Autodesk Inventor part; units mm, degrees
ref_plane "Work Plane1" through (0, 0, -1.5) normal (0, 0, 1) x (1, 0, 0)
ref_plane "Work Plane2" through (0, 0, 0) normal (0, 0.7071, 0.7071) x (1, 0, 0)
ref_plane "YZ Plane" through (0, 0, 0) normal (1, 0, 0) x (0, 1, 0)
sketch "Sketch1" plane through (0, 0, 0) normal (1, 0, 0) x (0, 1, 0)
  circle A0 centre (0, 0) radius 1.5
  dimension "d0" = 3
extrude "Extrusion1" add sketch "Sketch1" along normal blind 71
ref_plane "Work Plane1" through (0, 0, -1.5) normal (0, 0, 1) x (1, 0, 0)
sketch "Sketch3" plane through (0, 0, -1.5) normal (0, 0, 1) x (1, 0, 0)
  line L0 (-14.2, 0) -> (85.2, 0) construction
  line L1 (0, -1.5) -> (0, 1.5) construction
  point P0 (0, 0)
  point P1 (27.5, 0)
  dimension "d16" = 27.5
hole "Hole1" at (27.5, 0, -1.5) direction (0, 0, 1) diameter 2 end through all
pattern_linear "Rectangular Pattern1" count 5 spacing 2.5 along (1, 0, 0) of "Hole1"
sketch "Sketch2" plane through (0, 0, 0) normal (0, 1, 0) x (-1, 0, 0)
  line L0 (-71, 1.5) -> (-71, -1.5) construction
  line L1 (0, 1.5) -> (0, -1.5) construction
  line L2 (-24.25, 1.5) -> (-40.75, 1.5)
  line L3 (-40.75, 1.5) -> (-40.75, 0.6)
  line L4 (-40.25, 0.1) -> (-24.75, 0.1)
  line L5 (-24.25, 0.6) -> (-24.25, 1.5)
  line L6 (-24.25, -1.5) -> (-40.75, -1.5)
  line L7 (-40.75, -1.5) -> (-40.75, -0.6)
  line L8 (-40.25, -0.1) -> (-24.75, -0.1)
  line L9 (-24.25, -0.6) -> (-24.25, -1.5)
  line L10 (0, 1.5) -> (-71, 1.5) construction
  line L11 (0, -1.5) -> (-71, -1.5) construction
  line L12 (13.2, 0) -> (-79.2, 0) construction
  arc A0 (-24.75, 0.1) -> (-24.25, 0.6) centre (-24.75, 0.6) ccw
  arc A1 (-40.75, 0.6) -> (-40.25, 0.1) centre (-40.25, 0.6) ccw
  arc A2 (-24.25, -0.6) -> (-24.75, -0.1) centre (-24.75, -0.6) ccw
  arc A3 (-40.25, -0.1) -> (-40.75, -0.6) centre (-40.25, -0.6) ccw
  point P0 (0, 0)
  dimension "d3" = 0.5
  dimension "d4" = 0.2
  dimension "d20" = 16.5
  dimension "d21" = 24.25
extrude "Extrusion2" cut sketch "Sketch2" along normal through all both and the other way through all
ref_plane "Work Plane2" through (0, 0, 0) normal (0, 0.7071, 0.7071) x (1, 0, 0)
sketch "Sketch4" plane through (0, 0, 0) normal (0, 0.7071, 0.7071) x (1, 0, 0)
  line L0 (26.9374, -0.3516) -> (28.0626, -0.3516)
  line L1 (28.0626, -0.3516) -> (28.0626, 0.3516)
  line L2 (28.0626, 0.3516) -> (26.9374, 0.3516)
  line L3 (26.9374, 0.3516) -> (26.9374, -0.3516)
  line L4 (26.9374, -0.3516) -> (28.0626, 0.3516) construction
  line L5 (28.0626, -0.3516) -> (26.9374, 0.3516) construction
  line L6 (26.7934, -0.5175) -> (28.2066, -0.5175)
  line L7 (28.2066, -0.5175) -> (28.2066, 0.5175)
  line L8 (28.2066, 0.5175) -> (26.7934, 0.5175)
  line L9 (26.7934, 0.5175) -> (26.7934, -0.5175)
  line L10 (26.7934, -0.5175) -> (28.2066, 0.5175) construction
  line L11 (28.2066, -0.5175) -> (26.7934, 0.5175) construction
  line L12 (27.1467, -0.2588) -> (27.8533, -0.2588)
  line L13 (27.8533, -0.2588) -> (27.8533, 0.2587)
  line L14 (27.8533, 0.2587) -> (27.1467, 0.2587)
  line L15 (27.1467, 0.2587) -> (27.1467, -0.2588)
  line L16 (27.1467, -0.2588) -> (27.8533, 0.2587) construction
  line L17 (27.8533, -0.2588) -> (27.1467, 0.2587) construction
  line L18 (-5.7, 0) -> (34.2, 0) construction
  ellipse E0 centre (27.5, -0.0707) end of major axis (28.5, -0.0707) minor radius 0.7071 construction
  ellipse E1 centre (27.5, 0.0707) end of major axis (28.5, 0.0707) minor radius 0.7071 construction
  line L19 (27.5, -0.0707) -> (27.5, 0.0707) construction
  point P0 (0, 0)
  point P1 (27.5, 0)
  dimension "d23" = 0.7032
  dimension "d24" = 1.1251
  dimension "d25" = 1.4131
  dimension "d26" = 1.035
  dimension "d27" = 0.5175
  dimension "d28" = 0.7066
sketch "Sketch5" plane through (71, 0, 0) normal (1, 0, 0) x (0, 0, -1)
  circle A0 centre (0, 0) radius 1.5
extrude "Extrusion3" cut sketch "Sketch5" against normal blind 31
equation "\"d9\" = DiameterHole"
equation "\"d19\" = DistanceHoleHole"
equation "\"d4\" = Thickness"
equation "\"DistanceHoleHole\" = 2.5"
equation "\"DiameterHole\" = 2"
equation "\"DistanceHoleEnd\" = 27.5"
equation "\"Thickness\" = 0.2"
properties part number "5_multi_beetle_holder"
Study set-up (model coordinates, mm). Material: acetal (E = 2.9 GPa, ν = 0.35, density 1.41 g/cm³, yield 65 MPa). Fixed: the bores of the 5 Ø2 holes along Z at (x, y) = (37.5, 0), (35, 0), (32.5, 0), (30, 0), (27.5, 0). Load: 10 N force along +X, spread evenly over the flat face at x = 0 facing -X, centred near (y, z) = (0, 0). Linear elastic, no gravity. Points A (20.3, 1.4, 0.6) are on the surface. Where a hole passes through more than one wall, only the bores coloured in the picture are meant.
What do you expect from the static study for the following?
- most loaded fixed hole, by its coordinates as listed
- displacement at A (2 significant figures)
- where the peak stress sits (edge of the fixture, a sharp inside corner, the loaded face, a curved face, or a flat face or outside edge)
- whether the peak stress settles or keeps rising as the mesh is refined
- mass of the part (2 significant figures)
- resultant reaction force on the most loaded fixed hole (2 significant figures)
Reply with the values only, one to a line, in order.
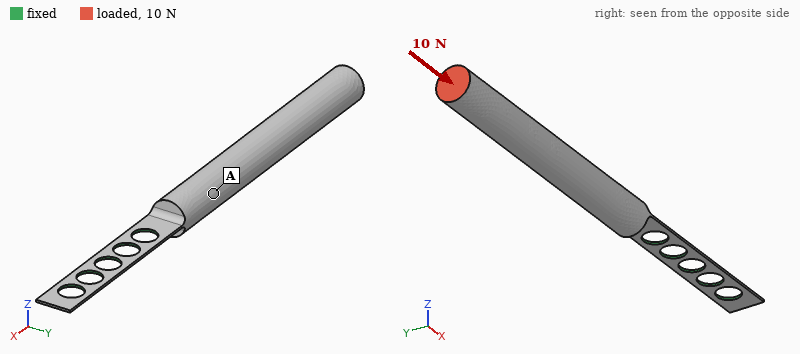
(27.5, 0)
17 µm
edge of the fixture
keeps rising
0.25 g
9.8 N
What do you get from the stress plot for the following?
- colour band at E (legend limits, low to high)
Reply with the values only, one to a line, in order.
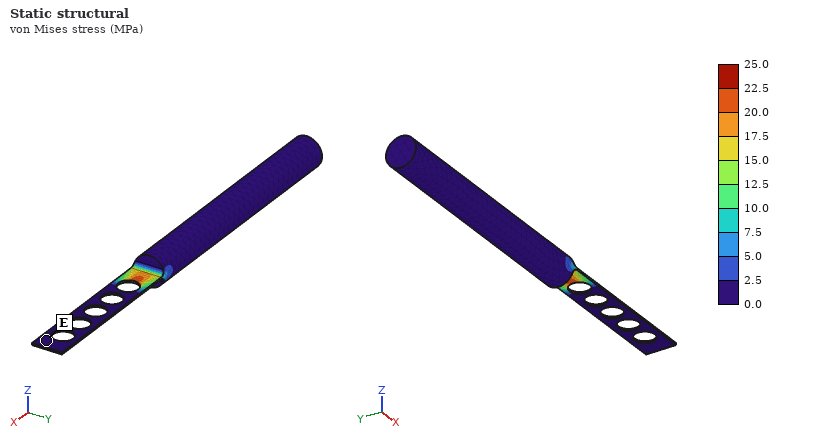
0.0 to 2.5 MPa
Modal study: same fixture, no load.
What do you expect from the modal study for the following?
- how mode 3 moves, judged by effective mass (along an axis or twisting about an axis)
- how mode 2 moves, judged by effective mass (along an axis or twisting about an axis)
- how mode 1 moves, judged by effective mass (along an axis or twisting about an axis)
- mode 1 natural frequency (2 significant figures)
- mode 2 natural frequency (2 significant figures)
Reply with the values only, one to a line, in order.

twisting about X
along Y
along Z
37 Hz
410 Hz
